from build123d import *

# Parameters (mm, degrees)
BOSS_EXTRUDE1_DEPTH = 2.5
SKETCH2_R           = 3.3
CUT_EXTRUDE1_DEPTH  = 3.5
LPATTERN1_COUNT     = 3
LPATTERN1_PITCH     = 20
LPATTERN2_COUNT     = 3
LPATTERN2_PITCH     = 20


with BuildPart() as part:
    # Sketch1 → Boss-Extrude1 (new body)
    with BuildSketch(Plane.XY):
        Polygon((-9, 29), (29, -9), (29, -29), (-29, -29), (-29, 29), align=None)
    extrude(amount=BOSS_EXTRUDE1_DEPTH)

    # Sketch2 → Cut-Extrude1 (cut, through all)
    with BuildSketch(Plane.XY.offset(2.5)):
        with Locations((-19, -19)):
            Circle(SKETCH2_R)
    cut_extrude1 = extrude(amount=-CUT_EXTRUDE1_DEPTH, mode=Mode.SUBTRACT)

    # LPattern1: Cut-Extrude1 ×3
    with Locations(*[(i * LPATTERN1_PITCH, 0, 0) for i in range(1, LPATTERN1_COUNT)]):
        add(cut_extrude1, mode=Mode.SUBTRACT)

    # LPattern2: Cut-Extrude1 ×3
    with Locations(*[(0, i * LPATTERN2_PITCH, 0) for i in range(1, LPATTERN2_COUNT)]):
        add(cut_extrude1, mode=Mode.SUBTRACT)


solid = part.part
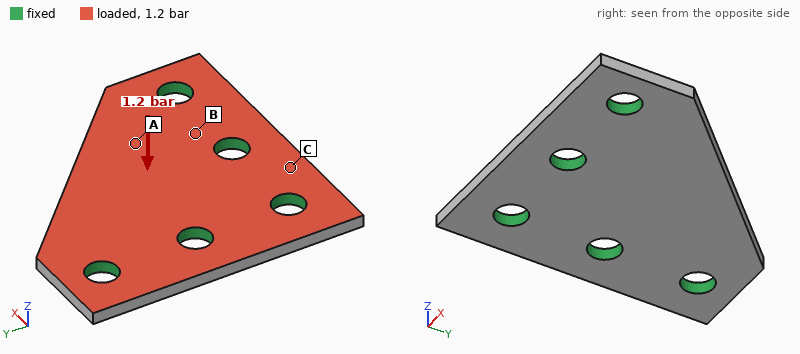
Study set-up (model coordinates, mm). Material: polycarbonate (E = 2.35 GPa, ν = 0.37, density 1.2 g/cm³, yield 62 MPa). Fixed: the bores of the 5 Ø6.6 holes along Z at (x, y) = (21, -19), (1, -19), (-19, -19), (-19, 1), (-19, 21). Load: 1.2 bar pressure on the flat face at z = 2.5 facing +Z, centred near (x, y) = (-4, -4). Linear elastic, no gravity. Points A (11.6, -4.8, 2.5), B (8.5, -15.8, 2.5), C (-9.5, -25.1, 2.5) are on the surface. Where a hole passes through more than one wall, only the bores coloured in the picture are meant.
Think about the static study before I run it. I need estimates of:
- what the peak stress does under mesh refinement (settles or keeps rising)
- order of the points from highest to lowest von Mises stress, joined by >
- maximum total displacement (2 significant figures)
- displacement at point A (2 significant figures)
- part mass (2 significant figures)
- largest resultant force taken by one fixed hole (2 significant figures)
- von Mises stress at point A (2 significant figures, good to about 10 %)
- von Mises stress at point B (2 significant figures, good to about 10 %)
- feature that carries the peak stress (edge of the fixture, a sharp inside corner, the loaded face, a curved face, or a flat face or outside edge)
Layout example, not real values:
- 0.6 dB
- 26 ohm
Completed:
- keeps rising
- B > A > C
- 0.76 mm
- 0.30 mm
- 7.4 g
- 66 N
- 4.6 MPa
- 8.0 MPa
- edge of the fixture
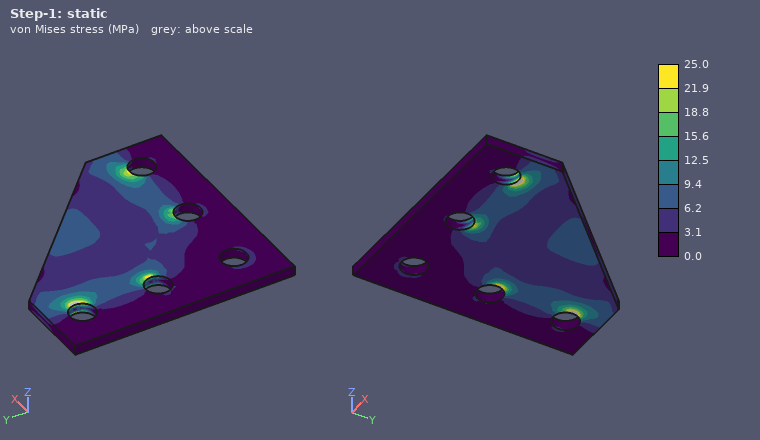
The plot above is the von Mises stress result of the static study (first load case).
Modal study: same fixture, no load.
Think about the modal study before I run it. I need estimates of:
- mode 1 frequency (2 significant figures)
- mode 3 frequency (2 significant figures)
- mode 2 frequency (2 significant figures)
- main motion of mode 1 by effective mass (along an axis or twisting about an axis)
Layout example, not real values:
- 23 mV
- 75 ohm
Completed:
- 1600 Hz
- 4900 Hz
- 3400 Hz
- along Z
